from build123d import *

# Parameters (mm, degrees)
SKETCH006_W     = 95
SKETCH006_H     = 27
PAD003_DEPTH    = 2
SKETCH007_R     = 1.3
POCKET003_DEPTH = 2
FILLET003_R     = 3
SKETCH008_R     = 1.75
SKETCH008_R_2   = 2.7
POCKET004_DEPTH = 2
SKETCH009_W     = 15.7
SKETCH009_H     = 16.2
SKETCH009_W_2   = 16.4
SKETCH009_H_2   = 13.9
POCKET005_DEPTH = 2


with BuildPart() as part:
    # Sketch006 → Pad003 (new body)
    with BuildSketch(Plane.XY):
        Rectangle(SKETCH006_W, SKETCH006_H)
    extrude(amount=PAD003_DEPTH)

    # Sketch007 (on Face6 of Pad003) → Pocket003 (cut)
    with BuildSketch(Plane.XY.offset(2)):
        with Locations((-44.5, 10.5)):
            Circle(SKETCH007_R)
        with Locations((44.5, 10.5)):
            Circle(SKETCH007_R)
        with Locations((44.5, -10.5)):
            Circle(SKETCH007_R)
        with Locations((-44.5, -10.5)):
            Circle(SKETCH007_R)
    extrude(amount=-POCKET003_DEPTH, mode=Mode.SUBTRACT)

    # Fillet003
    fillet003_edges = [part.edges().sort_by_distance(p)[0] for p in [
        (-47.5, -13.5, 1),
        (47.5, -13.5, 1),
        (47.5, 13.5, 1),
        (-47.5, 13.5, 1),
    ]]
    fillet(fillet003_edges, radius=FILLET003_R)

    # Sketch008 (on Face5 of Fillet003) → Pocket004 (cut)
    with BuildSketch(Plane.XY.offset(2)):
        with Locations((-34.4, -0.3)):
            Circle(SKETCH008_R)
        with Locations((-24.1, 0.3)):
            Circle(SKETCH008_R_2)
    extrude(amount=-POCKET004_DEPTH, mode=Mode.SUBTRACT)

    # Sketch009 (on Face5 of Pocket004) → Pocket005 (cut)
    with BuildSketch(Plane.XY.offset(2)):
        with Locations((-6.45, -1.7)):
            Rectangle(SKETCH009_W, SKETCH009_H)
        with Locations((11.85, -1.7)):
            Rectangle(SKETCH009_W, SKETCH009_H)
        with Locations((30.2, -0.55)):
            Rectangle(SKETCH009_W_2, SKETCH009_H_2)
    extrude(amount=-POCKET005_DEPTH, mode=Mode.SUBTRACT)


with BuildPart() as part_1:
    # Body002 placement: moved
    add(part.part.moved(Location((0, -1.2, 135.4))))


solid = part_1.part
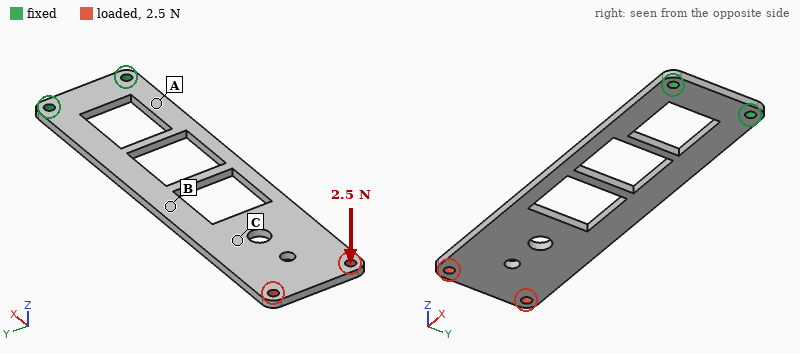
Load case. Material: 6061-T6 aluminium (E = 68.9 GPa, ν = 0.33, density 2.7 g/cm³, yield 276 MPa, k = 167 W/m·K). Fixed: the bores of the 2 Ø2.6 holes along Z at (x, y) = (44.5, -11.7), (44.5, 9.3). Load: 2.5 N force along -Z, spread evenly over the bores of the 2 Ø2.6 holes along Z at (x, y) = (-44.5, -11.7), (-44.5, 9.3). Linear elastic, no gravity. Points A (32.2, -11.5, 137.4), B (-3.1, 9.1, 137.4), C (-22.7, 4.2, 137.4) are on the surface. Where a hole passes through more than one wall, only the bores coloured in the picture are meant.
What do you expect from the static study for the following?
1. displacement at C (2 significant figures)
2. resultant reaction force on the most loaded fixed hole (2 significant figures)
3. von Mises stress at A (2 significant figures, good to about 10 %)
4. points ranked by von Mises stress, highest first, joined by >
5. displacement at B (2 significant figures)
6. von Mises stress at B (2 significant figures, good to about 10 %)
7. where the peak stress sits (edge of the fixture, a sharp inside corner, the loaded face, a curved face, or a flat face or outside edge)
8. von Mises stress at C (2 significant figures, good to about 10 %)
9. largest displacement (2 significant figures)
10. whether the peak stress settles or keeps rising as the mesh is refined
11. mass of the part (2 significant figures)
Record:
0.63 mm
1.3 N
21 MPa
A > B > C
0.33 mm
14 MPa
edge of the fixture
4.0 MPa
1.0 mm
keeps rising
9.5 g
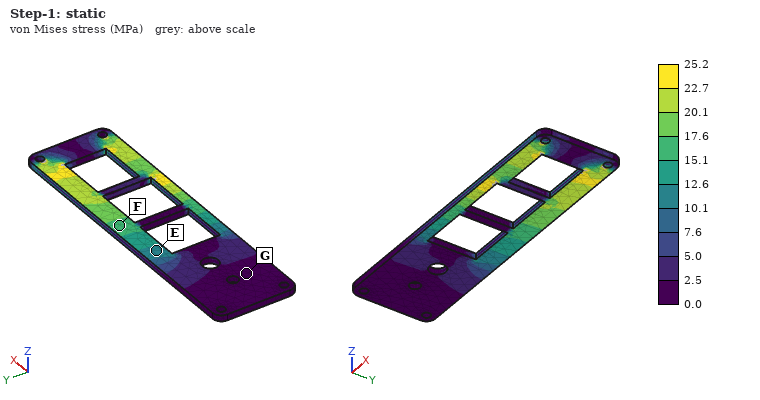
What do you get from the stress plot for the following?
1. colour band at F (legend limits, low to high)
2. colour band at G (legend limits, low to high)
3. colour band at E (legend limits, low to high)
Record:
15.1 to 17.6 MPa
0.0 to 2.5 MPa
10.1 to 12.6 MPa
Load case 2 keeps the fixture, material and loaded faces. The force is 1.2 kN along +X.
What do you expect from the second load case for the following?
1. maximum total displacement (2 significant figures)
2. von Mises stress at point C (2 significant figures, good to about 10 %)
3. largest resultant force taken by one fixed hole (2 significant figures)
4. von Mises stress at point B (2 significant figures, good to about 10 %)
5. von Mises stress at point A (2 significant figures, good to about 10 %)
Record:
0.11 mm
25 MPa
610 N
45 MPa
46 MPa
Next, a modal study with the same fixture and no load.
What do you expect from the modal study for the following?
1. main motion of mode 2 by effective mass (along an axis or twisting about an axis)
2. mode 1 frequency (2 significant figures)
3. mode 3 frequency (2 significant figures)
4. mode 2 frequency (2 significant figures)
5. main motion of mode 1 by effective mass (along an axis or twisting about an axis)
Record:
twisting about X
140 Hz
1100 Hz
930 Hz
along Z
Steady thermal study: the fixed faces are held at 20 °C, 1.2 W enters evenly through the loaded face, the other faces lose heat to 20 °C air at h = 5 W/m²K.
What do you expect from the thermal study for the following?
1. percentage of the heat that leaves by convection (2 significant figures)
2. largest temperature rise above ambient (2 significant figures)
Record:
20 %
20 K
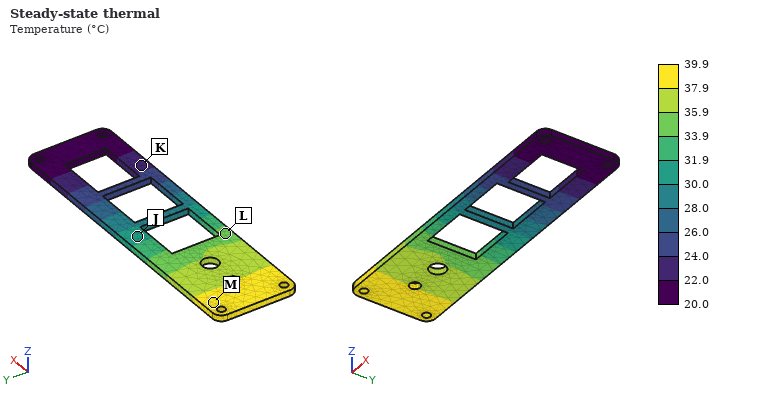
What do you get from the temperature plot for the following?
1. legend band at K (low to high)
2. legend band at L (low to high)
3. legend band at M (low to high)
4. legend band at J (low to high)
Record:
22.0 to 24.0 °C
33.9 to 35.9 °C
37.9 to 39.9 °C
30.0 to 31.9 °C
